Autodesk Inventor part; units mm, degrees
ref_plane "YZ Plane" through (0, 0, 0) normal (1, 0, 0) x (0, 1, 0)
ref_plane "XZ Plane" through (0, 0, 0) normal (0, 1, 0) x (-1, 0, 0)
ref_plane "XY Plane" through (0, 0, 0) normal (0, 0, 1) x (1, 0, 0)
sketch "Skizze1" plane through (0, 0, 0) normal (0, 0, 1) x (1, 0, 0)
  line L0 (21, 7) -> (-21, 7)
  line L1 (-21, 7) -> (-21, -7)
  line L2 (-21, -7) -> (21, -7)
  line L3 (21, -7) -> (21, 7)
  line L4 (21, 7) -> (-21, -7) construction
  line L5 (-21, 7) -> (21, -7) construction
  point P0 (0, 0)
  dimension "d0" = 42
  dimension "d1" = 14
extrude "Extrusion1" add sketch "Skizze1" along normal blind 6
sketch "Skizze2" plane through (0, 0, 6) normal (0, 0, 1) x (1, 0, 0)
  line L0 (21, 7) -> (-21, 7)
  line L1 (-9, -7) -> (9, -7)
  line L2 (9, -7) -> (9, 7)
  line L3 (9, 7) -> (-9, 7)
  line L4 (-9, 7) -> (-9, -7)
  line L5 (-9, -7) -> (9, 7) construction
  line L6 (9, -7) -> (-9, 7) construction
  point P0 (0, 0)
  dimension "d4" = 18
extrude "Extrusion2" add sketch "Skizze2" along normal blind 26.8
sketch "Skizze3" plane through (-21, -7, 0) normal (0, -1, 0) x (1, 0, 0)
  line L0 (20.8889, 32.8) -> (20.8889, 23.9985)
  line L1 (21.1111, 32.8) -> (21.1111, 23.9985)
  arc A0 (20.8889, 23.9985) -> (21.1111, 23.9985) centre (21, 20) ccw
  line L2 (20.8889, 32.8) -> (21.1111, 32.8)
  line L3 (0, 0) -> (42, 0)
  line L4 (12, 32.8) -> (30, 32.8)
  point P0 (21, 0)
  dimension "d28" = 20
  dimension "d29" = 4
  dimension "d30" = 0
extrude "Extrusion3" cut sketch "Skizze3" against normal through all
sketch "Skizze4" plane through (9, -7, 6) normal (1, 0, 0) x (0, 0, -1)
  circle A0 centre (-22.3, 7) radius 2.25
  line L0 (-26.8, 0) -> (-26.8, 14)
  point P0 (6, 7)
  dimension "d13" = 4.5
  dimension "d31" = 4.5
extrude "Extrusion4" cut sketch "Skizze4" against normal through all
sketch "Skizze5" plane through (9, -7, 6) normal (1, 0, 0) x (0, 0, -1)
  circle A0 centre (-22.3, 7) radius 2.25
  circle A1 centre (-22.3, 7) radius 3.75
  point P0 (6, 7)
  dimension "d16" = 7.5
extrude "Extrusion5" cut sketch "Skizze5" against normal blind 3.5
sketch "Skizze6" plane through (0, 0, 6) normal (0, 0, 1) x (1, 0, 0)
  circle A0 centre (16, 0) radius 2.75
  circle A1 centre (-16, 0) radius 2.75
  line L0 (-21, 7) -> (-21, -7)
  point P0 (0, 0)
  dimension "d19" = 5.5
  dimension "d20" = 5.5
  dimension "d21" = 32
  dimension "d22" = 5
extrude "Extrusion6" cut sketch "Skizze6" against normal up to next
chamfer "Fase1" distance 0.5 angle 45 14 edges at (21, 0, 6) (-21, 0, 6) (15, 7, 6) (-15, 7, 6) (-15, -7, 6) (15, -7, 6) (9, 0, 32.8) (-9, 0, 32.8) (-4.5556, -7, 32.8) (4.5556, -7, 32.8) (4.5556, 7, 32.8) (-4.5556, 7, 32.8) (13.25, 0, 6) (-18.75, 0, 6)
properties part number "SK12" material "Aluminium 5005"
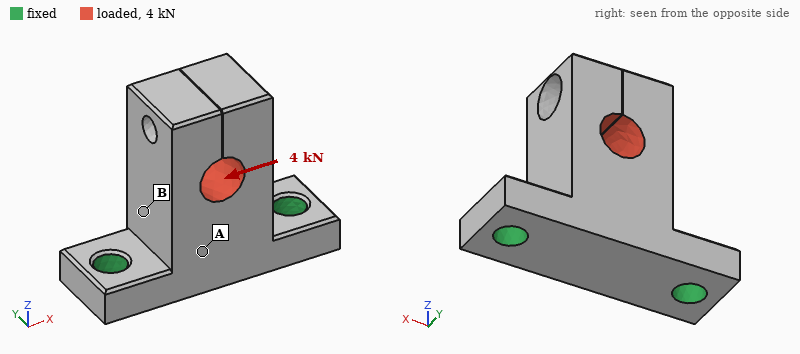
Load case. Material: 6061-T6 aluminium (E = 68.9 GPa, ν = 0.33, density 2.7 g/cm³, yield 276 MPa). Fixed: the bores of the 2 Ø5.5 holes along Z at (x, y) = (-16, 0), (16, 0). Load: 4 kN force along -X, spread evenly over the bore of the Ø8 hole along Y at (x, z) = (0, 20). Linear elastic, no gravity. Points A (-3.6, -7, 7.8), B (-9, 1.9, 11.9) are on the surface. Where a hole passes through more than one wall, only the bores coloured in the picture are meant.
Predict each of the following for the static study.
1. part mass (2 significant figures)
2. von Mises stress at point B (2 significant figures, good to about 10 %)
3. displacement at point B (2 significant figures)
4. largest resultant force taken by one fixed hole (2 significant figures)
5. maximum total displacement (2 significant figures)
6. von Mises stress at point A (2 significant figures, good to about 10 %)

24 g
63 MPa
0.031 mm
3.5 kN
0.12 mm
30 MPa
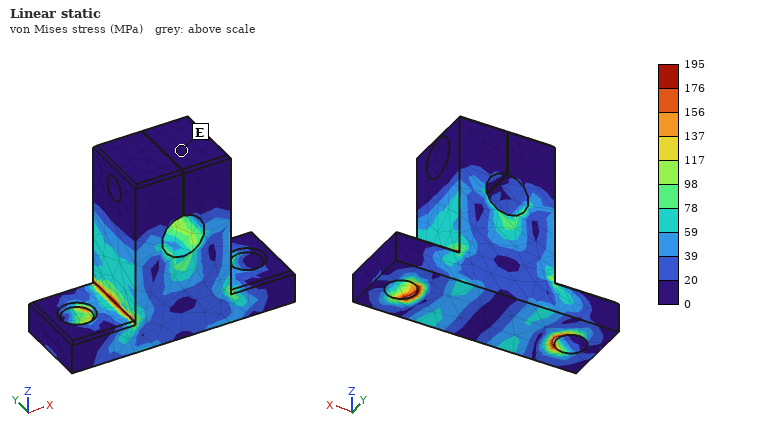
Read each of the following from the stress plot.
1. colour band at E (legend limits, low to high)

0 to 20 MPa
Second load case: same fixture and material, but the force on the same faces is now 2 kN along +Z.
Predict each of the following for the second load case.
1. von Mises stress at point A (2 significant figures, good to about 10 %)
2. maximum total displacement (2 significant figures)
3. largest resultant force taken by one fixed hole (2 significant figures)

12 MPa
29 µm
1.1 kN
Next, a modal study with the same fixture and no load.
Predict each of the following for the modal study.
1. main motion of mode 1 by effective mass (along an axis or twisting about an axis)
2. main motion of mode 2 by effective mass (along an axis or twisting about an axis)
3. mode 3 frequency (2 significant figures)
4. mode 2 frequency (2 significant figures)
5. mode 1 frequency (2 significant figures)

along Y
along X
10 kHz
8300 Hz
5100 Hz
